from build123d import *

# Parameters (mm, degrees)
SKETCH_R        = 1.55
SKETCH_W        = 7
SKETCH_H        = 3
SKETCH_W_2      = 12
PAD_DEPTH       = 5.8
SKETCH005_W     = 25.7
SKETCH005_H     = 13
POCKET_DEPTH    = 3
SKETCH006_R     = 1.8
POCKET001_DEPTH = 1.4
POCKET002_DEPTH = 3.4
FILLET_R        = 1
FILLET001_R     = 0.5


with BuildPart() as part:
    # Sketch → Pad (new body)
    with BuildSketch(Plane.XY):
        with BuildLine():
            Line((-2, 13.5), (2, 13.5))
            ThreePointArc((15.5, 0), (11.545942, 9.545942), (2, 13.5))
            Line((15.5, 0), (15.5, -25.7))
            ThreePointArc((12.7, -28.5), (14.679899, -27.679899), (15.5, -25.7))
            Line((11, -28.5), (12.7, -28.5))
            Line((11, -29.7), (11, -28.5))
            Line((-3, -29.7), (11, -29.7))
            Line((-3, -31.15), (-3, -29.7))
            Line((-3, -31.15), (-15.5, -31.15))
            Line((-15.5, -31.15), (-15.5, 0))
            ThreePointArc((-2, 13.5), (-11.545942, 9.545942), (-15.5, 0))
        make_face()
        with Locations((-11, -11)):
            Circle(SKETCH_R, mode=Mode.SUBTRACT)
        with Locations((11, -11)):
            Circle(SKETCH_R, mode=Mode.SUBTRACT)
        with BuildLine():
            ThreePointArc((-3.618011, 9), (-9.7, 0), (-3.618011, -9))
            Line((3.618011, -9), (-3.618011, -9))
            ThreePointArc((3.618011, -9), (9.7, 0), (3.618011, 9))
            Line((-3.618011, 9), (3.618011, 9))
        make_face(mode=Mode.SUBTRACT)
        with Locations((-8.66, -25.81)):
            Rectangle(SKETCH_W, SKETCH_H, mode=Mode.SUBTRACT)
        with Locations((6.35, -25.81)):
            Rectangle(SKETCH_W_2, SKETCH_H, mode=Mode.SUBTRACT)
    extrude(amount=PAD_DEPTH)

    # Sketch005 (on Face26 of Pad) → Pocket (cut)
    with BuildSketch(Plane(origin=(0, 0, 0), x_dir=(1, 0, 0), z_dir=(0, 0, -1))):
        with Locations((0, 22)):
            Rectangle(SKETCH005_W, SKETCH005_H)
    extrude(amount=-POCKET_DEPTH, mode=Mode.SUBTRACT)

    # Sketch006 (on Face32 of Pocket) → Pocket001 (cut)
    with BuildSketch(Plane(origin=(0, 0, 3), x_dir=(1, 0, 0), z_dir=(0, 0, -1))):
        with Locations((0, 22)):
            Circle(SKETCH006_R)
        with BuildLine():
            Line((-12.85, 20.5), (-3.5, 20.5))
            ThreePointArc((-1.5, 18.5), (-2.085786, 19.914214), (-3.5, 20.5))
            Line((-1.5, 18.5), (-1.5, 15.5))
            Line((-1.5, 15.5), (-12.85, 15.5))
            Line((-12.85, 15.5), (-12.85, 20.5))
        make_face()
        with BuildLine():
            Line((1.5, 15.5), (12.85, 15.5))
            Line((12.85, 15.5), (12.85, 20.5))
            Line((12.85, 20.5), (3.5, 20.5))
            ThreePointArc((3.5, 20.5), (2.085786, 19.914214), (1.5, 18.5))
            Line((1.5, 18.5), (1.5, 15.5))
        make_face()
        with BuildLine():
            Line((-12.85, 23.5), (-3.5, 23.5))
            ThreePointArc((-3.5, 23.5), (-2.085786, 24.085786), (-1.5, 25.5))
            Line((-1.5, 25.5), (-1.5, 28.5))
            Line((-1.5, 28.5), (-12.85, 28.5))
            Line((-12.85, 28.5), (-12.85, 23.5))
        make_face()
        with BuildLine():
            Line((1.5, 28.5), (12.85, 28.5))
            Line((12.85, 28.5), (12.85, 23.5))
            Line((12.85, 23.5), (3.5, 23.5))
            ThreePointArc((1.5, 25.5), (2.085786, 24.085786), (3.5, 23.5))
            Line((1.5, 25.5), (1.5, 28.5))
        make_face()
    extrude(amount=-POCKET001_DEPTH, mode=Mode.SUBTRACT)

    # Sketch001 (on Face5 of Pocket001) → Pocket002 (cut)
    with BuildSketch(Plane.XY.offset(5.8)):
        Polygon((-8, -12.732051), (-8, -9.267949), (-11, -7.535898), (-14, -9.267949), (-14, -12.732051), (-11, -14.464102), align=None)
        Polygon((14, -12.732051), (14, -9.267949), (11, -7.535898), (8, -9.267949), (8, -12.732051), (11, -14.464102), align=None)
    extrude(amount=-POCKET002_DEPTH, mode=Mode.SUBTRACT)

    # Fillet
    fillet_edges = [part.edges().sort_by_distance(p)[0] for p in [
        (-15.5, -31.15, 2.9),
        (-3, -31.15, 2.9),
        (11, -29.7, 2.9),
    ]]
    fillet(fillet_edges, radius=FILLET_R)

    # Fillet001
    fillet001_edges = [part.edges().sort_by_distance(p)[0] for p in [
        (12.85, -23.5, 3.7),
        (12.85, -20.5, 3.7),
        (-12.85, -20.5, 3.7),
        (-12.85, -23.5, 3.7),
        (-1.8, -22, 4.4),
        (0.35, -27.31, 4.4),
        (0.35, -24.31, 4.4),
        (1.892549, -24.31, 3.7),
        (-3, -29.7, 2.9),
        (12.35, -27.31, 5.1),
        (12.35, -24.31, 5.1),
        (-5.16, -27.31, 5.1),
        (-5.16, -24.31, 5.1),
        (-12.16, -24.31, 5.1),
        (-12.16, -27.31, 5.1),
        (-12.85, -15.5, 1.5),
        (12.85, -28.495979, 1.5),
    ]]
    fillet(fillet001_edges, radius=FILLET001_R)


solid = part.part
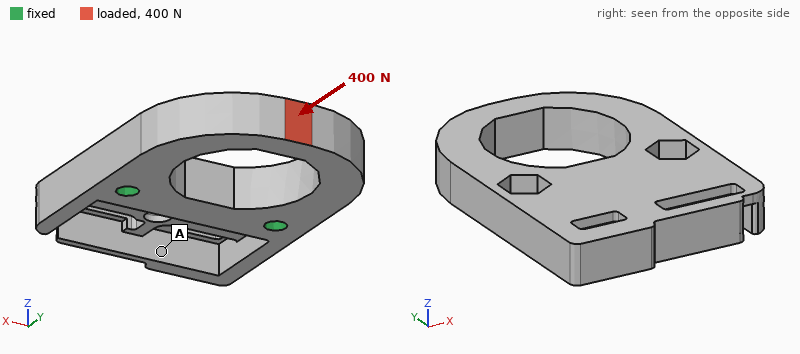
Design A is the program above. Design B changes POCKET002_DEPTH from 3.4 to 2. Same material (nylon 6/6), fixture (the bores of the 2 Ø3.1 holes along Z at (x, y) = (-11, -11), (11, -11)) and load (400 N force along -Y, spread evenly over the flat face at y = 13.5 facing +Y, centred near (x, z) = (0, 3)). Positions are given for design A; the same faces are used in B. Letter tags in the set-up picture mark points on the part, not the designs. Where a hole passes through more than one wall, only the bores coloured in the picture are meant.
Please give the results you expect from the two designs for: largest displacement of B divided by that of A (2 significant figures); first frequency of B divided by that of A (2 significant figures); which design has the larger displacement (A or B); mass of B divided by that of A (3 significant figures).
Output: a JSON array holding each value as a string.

["0.70", "1.3", "A", "1.02"]
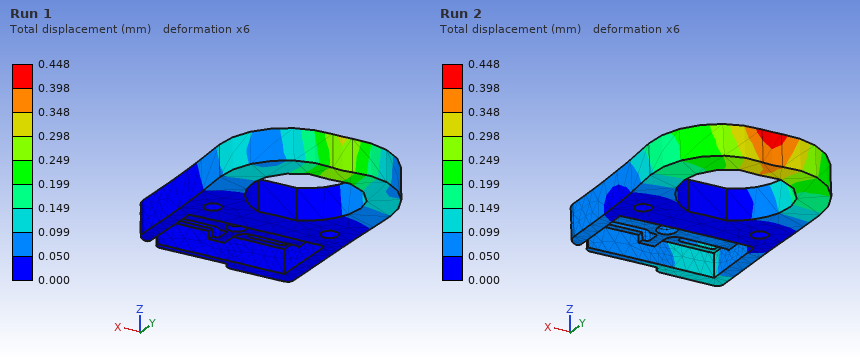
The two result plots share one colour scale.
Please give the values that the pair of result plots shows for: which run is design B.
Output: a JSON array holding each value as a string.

["Run 1"]
